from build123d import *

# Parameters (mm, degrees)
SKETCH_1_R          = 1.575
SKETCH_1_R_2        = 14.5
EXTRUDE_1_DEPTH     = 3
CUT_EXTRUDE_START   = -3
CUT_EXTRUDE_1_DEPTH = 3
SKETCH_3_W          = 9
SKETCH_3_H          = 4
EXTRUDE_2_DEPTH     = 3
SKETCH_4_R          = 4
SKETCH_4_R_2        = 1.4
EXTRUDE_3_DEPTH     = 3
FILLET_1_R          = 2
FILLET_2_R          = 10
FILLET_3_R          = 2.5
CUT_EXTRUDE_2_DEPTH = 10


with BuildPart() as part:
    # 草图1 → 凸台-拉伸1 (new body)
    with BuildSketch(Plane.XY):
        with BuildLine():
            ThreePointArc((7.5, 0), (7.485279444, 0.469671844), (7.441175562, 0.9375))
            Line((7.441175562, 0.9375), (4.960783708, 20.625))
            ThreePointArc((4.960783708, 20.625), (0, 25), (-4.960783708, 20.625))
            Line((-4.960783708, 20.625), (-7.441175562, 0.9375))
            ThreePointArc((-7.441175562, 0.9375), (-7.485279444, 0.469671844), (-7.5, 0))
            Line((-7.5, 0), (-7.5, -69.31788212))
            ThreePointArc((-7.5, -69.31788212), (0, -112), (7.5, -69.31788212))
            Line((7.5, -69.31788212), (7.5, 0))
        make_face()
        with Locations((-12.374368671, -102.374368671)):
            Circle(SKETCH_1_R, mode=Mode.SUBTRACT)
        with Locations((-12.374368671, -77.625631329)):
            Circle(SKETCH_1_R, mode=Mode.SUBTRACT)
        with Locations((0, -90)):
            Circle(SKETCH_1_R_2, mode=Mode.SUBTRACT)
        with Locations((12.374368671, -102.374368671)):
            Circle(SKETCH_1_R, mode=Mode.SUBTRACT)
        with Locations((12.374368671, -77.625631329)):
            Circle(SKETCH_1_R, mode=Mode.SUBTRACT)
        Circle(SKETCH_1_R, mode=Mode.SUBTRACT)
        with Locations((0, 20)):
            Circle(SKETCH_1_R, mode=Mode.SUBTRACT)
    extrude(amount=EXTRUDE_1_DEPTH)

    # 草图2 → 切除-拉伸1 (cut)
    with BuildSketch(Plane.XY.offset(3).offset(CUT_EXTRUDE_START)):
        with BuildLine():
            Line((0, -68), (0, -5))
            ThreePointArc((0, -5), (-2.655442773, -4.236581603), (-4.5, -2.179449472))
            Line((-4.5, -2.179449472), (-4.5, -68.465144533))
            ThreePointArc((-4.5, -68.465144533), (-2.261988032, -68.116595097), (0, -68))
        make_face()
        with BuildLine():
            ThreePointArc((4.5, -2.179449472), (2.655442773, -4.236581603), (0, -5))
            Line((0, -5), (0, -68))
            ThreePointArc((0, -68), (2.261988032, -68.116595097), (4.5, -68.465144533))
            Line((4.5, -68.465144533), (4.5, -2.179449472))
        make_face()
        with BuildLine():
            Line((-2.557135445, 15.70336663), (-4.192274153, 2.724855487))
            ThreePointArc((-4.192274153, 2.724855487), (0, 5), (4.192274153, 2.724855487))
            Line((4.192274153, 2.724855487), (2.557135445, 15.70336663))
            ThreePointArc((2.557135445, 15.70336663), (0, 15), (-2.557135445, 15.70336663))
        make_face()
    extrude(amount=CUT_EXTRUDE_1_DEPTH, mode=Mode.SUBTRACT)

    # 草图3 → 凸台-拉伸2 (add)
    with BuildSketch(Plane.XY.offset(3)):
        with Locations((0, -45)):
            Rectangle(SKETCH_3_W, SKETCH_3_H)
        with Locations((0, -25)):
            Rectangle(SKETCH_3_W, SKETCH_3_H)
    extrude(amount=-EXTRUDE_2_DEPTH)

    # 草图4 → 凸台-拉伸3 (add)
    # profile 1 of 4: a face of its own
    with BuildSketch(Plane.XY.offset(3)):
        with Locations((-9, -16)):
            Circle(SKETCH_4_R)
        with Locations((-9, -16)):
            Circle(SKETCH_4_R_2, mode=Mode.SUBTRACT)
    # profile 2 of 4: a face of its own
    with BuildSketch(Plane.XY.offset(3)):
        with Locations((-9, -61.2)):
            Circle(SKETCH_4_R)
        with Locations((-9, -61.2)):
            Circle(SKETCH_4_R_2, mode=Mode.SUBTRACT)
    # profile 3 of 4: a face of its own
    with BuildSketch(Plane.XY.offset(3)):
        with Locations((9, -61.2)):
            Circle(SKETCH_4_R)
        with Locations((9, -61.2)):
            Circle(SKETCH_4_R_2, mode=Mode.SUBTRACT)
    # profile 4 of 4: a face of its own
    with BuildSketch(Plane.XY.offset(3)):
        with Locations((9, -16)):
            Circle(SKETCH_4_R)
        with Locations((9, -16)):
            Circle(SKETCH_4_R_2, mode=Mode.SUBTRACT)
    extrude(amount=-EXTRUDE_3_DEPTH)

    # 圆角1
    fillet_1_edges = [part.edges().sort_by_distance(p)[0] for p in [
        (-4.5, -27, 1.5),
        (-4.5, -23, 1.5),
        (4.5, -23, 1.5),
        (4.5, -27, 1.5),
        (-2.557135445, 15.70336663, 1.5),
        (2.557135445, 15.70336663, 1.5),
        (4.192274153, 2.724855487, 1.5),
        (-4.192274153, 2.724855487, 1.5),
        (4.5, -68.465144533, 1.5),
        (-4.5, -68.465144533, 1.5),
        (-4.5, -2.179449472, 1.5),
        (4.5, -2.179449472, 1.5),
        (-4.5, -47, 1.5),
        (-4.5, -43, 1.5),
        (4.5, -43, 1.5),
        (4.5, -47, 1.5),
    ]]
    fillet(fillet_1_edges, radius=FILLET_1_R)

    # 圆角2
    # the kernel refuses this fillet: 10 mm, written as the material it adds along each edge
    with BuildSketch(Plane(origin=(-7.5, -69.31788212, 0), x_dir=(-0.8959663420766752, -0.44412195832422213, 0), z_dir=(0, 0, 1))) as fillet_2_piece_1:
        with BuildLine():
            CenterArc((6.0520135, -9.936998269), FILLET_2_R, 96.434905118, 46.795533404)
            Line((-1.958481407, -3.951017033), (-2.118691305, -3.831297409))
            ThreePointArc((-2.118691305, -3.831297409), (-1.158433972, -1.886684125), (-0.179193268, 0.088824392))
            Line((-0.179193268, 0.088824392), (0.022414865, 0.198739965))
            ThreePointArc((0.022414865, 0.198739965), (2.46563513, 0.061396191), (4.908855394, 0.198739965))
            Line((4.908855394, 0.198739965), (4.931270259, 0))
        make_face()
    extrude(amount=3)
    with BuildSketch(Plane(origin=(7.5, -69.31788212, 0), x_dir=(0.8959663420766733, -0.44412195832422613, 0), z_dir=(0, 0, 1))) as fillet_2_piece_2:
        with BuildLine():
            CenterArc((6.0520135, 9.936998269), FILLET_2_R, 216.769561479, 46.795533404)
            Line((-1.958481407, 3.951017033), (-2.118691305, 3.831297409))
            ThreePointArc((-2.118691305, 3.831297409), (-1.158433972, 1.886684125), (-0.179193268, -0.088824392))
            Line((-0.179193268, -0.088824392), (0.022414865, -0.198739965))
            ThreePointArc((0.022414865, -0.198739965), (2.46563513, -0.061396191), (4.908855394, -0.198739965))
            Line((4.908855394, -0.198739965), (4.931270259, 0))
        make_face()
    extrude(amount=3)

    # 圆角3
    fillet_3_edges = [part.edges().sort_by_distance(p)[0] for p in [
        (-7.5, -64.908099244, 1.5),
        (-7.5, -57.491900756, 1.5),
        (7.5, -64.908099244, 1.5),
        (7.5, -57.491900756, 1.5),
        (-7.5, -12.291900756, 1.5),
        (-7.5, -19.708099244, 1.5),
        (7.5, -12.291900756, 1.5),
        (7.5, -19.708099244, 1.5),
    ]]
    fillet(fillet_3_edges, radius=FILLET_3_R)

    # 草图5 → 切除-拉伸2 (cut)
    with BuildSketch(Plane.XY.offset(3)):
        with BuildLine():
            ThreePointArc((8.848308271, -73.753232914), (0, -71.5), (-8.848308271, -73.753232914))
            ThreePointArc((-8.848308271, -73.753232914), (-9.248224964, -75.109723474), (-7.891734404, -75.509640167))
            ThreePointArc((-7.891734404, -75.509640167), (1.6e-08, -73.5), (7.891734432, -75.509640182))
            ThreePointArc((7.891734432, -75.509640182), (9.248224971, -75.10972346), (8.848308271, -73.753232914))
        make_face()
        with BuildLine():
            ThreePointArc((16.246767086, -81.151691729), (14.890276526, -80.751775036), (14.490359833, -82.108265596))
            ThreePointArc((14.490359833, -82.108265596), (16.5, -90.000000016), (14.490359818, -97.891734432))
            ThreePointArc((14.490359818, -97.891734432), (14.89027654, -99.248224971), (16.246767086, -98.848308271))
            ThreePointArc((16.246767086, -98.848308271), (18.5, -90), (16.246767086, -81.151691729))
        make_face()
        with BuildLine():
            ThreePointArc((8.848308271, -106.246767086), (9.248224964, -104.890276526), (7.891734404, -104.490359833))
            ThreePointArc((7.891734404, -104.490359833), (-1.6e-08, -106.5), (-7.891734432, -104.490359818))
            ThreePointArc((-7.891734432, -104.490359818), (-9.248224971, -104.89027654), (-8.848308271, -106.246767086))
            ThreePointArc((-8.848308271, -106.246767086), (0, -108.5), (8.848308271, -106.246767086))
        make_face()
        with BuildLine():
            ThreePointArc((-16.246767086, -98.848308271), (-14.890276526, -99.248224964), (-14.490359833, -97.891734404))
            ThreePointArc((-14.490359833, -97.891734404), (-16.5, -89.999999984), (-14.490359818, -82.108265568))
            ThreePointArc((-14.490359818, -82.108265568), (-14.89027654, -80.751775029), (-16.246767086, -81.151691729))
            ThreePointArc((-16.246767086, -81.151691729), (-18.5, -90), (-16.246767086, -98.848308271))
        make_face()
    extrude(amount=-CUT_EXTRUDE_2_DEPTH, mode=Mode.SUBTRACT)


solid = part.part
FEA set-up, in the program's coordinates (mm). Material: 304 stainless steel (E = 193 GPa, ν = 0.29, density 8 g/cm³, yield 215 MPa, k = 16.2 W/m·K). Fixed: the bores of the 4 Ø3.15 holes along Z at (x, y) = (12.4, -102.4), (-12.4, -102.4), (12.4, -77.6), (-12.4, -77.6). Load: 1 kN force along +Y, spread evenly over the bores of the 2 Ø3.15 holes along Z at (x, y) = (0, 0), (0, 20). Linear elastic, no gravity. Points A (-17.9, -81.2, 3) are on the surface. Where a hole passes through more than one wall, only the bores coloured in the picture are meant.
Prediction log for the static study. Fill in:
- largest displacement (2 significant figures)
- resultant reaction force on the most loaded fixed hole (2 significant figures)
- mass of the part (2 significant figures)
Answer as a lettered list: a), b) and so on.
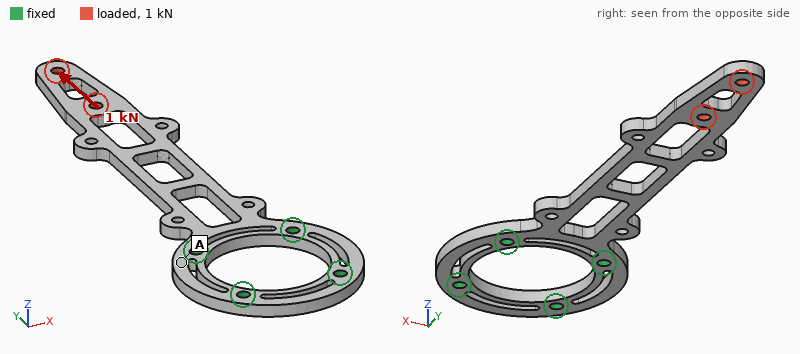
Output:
a) 25 µm
b) 580 N
c) 38 g
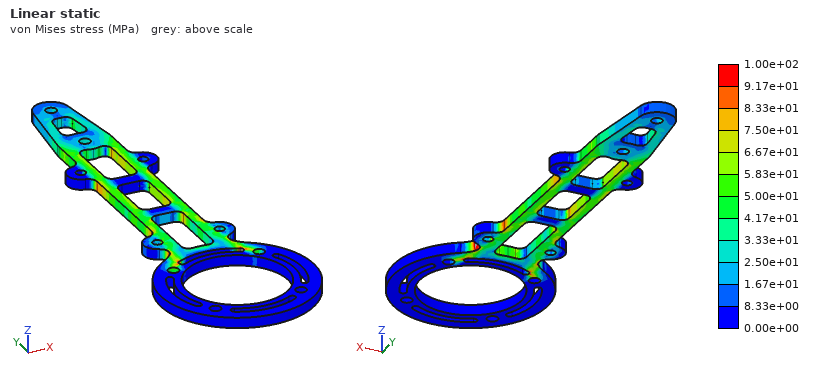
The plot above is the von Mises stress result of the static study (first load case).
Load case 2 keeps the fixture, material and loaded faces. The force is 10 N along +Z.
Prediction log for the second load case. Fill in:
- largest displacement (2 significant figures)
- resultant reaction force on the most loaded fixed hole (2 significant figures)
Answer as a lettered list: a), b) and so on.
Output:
a) 0.87 mm
b) 5.3 N
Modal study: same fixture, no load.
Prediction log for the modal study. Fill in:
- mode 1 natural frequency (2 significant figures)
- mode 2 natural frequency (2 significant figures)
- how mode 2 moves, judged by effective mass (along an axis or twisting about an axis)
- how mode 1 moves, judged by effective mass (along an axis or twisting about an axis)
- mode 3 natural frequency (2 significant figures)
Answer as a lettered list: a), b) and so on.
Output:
a) 210 Hz
b) 1200 Hz
c) along X
d) along Z
e) 1300 Hz
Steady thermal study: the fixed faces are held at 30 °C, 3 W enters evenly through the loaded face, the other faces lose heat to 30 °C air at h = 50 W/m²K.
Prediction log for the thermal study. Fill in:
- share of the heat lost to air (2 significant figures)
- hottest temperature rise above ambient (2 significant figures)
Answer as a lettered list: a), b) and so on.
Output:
a) 100 %
b) 70 K
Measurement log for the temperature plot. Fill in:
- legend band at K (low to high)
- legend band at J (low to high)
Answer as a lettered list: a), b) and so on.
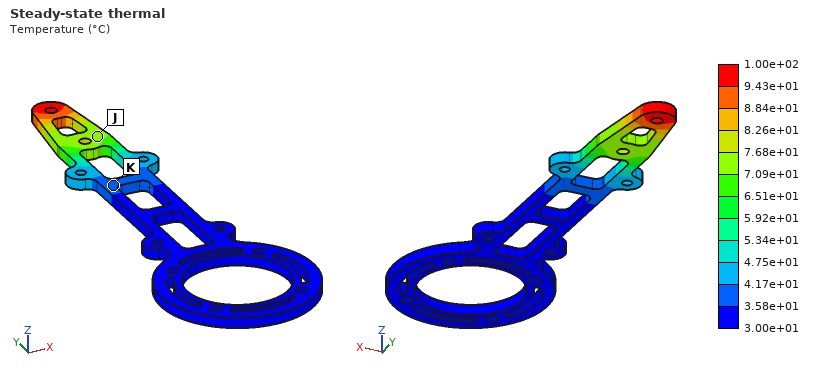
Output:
a) 3.58e+01 to 4.17e+01 °C
b) 7.09e+01 to 7.68e+01 °C
